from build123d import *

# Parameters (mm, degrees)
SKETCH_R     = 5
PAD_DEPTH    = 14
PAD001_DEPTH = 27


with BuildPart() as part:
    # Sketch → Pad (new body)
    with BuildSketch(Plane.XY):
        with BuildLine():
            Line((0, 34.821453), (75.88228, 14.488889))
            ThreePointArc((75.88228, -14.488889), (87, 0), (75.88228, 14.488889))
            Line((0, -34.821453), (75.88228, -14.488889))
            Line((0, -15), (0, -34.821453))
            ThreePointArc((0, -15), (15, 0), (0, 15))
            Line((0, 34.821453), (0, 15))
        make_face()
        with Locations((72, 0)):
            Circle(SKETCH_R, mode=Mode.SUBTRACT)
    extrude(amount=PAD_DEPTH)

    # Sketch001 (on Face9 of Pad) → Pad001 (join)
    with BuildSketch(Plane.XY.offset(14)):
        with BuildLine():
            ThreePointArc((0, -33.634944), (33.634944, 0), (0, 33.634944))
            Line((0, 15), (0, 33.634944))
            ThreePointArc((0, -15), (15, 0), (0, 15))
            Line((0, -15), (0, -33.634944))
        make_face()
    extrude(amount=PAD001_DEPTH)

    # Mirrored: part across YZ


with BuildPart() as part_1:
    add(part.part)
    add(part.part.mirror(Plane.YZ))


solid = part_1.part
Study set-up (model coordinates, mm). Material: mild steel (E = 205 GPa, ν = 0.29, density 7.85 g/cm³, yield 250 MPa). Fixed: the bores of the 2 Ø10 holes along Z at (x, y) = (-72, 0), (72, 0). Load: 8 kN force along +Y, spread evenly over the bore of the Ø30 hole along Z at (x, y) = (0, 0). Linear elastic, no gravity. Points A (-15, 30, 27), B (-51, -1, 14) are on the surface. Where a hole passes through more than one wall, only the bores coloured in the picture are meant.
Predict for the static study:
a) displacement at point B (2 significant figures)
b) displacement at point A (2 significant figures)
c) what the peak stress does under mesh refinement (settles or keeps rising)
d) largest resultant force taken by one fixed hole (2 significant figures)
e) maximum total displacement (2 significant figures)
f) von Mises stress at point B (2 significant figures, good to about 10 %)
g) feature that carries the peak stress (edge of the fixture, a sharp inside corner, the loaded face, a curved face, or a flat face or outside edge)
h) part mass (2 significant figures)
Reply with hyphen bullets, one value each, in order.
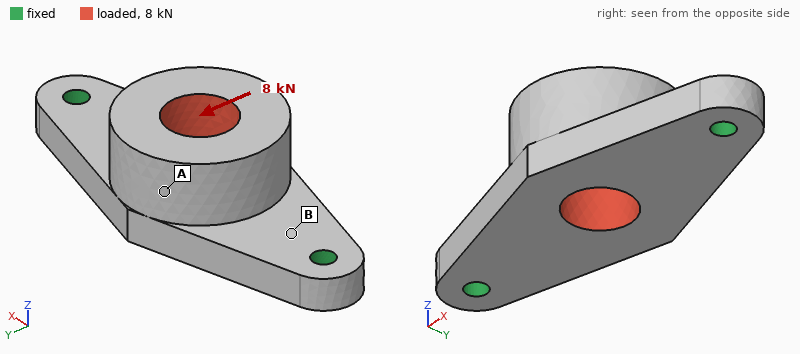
- 8.0 µm
- 39 µm
- keeps rising
- 4.0 kN
- 51 µm
- 52 MPa
- edge of the fixture
- 1.4 kg
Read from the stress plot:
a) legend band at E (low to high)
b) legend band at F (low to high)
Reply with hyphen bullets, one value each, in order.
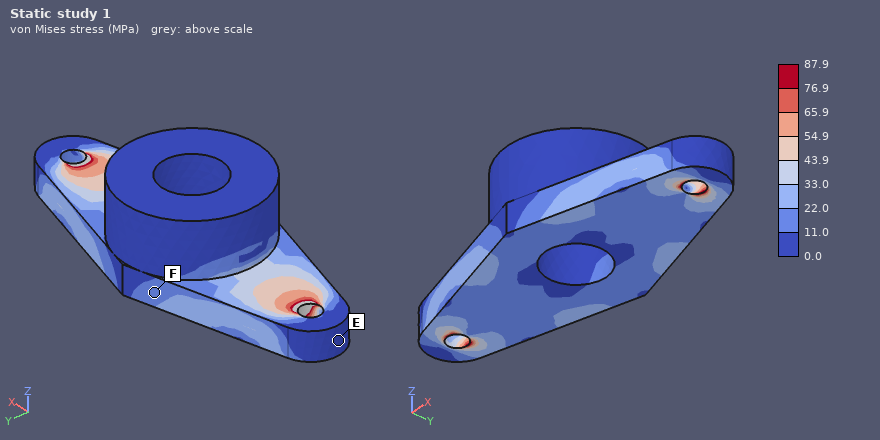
- 0.0 to 11.0 MPa
- 11.0 to 22.0 MPa
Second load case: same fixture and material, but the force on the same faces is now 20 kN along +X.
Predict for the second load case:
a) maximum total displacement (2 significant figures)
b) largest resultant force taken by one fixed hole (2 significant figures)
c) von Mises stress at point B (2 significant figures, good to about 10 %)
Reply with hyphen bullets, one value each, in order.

- 16 µm
- 10 kN
- 29 MPa
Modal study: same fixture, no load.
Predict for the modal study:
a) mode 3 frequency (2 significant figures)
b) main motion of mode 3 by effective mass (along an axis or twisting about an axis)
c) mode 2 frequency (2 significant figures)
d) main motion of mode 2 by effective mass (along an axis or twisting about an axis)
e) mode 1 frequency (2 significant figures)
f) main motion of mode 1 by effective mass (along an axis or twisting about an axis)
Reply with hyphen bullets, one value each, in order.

- 5300 Hz
- along Y
- 2800 Hz
- along Z
- 2100 Hz
- along Y
